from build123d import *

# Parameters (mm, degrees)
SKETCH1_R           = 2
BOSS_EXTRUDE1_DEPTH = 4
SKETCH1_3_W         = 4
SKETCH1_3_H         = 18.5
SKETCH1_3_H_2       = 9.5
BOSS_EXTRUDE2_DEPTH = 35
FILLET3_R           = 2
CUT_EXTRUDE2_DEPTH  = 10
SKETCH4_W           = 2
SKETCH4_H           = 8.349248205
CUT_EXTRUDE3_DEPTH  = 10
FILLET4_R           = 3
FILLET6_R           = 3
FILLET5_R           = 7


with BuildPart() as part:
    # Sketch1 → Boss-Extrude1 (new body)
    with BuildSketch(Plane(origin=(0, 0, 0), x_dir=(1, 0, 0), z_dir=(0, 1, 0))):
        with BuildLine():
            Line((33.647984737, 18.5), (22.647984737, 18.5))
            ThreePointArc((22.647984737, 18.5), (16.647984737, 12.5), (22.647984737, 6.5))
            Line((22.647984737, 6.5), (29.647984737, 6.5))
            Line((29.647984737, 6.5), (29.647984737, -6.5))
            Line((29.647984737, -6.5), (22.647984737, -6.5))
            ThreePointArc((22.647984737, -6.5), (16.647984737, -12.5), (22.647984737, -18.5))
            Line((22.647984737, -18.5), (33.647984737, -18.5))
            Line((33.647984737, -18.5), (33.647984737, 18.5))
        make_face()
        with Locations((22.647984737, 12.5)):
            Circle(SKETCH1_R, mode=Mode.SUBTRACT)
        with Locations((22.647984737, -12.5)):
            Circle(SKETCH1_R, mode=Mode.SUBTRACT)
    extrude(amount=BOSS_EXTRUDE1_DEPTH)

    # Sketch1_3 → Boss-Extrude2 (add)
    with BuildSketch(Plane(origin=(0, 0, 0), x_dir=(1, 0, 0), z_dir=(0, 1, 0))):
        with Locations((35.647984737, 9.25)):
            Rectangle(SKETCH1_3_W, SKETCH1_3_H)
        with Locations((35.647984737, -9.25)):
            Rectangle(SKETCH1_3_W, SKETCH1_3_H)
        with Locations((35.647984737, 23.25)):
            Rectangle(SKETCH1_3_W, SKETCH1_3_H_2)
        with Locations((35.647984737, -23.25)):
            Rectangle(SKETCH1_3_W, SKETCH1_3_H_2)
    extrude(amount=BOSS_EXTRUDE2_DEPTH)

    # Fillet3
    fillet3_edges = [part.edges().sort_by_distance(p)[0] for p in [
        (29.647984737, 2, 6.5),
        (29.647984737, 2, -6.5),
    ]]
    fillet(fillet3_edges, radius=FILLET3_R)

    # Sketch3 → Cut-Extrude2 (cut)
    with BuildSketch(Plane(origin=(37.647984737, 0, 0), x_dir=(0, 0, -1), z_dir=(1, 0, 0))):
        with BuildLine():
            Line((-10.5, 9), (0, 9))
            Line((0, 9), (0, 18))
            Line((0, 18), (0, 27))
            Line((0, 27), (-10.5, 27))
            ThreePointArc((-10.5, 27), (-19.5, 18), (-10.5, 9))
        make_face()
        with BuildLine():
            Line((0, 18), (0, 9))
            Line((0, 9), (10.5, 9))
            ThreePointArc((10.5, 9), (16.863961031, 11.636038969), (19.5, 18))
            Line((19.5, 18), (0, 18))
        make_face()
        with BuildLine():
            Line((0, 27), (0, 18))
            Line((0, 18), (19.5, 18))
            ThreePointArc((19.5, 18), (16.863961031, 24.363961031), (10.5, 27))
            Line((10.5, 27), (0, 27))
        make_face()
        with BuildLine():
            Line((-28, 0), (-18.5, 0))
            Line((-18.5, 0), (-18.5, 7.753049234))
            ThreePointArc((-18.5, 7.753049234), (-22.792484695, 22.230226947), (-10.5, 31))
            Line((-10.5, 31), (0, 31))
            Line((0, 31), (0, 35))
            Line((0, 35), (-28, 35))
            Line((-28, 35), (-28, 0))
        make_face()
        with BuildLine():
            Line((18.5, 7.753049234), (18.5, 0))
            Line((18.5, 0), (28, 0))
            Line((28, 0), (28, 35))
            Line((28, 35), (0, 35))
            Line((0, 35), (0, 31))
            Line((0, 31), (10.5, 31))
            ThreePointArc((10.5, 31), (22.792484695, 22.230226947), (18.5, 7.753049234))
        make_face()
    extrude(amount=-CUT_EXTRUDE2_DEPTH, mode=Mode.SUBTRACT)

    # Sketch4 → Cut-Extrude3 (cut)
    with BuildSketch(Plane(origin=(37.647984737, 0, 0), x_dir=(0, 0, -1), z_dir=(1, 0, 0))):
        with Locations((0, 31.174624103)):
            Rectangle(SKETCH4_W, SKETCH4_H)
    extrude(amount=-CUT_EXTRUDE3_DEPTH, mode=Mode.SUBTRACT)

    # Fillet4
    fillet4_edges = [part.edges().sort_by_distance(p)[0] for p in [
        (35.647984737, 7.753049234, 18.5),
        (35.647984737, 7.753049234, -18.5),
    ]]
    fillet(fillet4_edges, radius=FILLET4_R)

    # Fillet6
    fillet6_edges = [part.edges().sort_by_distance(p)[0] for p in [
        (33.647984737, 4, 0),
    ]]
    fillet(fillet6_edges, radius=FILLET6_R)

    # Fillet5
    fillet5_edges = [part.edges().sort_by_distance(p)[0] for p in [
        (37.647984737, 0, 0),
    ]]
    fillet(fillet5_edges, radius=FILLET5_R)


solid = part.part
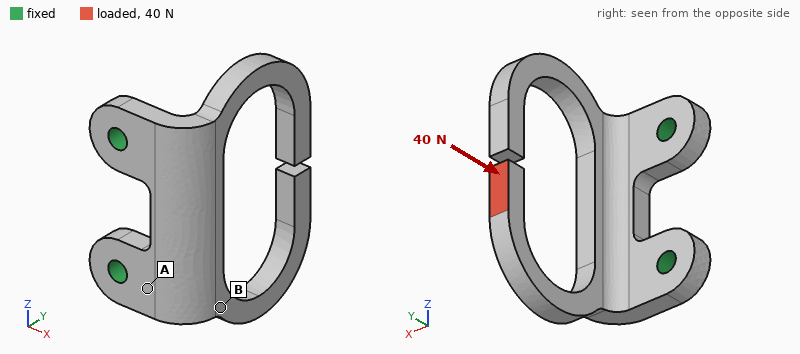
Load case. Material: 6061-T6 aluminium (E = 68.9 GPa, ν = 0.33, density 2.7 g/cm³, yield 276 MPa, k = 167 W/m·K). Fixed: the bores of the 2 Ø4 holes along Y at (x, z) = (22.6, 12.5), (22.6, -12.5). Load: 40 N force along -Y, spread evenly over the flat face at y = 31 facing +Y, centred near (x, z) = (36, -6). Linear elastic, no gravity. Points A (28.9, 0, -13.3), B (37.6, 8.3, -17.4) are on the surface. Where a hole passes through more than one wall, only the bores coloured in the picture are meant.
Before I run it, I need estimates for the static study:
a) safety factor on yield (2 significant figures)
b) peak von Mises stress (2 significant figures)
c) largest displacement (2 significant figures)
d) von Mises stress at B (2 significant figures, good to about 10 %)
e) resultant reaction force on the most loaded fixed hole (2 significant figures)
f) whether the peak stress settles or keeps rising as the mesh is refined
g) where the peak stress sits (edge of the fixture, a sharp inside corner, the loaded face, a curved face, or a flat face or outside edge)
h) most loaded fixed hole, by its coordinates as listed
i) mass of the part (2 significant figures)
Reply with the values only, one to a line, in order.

4.0
68 MPa
0.23 mm
16 MPa
29 N
settles
a curved face
(22.6, -12.5)
10 g
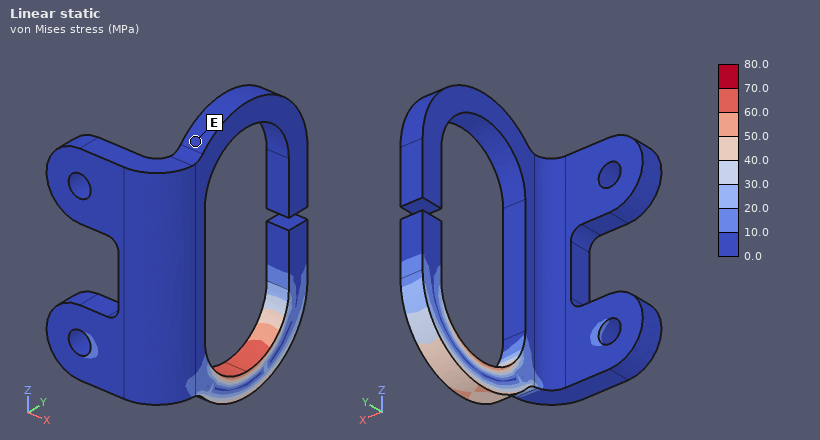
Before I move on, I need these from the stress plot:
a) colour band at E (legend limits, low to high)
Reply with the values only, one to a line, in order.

0.0 to 10.0 MPa
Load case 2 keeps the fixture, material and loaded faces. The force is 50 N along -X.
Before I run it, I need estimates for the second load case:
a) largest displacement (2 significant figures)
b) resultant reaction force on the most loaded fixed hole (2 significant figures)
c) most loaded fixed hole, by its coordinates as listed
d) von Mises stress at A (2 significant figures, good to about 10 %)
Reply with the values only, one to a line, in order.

0.65 mm
49 N
(22.6, -12.5)
30 MPa
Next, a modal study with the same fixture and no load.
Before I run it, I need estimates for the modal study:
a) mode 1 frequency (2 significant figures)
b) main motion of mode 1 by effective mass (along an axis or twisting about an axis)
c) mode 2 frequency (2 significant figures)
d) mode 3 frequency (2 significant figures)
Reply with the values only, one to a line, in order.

1900 Hz
along X
2000 Hz
2500 Hz
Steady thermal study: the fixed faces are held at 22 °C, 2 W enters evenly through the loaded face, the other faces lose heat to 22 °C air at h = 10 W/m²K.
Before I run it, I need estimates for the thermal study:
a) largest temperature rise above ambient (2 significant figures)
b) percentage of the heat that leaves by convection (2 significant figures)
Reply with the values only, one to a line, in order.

28 K
5.9 %
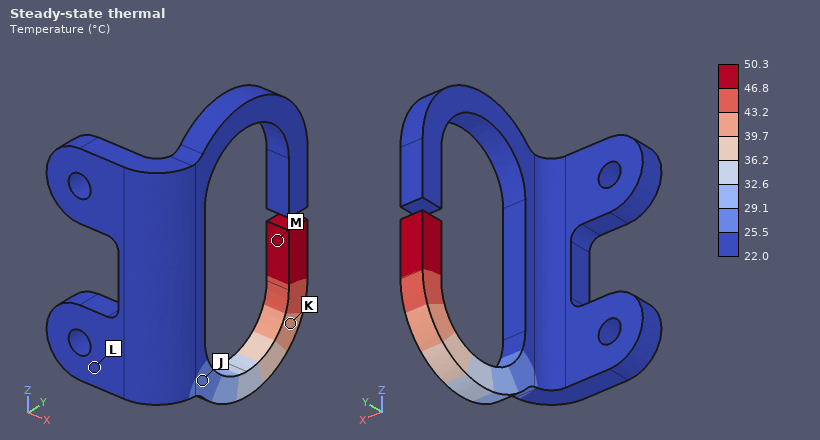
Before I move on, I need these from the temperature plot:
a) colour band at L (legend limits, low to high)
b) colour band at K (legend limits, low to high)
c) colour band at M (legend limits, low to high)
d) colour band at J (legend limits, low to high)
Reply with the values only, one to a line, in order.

22.0 to 25.5 °C
39.7 to 43.2 °C
46.8 to 50.3 °C
25.5 to 29.1 °C
